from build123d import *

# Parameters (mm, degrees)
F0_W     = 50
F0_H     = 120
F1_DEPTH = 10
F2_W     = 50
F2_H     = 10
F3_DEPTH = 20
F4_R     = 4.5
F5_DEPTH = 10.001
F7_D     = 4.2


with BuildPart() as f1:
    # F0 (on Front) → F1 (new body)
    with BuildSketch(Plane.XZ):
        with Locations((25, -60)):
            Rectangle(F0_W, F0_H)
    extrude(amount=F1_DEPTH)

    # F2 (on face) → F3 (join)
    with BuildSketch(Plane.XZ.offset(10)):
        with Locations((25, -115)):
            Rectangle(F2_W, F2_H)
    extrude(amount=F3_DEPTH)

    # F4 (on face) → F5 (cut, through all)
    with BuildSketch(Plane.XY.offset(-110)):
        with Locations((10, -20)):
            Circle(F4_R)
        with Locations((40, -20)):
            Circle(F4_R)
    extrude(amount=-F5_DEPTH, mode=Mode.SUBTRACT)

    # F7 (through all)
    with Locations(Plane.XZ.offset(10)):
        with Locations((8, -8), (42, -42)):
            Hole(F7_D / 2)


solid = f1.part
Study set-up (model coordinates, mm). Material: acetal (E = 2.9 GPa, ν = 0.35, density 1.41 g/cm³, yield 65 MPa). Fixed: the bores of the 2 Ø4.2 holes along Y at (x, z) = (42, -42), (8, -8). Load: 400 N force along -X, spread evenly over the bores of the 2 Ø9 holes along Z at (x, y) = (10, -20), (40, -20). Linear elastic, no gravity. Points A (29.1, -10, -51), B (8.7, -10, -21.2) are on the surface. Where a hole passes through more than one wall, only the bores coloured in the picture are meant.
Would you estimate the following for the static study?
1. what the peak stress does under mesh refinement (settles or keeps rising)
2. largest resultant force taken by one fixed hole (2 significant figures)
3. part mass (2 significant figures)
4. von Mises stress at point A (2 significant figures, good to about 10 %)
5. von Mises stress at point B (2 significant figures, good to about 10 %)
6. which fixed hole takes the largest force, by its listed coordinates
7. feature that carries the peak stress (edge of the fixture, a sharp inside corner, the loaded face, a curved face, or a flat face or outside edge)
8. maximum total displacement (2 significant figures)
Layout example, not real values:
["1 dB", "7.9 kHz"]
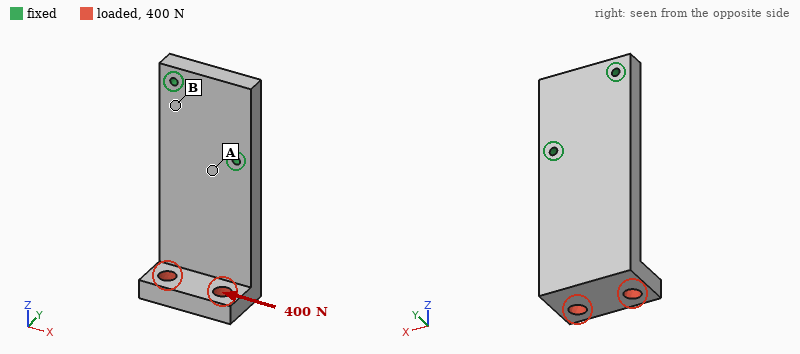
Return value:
["keeps rising", "870 N", "97 g", "8.3 MPa", "2.5 MPa", "(42, -42)", "edge of the fixture", "1.5 mm"]
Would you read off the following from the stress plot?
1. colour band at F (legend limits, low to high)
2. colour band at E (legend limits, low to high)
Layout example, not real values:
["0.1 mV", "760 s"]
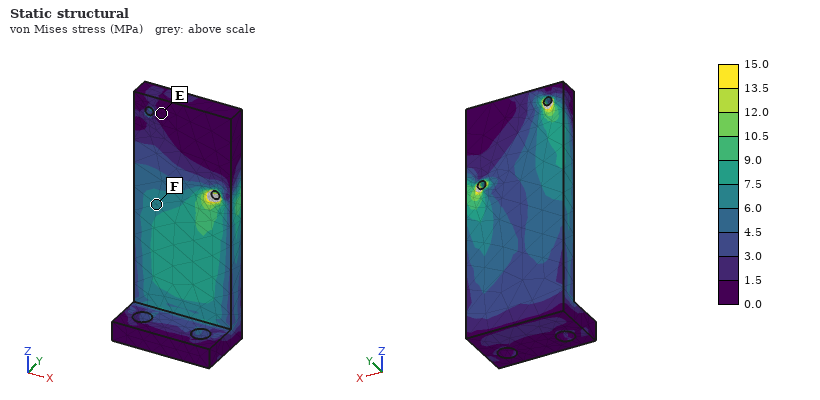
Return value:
["6.0 to 7.5 MPa", "0.0 to 1.5 MPa"]
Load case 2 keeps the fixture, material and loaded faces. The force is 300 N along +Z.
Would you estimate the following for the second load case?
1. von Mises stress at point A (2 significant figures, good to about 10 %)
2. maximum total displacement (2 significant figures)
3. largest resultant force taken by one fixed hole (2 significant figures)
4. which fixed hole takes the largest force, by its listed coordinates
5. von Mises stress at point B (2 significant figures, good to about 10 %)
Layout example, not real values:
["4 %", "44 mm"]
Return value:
["5.4 MPa", "1.6 mm", "180 N", "(42, -42)", "2.1 MPa"]
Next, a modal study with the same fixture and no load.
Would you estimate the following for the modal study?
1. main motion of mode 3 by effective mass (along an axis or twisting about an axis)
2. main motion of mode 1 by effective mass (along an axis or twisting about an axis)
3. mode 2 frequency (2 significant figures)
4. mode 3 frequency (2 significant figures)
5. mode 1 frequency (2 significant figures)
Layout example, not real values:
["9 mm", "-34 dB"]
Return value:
["along X", "along Y", "650 Hz", "980 Hz", "230 Hz"]
